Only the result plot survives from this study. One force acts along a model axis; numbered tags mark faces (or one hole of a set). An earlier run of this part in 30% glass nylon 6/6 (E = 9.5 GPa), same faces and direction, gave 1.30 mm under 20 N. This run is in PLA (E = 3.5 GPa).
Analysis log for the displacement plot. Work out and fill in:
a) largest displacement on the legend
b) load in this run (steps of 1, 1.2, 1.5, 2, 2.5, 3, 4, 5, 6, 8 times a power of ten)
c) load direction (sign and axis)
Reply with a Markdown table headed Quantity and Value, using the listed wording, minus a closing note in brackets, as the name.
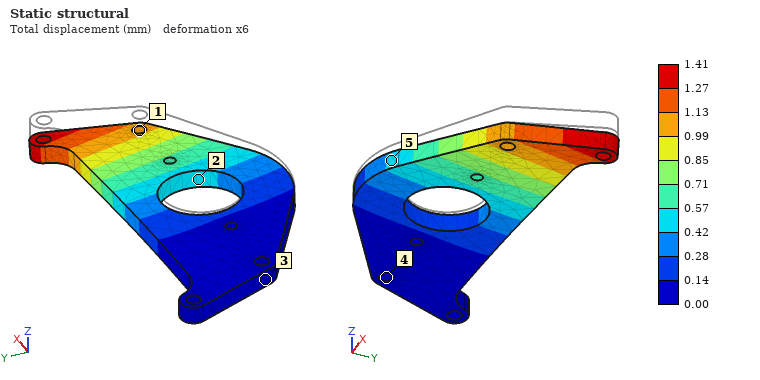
| Quantity | Value |
|---|---|
| largest displacement on the legend | 1.41 mm |
| load in this run | 8 N |
| load direction | -Z |
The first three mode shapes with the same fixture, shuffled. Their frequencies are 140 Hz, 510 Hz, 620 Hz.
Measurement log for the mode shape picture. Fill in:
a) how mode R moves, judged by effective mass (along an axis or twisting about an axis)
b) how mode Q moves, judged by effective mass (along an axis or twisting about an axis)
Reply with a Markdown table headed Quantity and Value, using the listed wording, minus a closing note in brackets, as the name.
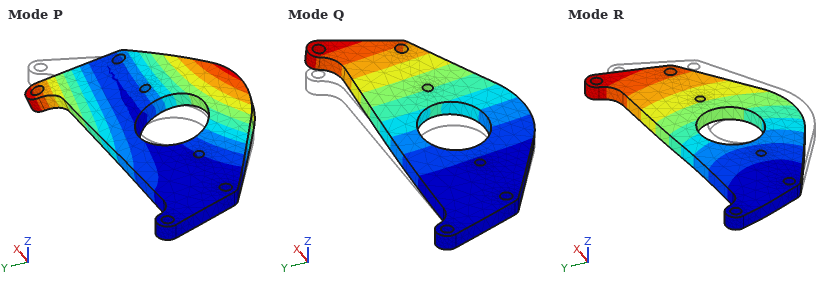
| Quantity | Value |
|---|---|
| how mode R moves, judged by effective mass | along Y |
| how mode Q moves, judged by effective mass | along Z |
